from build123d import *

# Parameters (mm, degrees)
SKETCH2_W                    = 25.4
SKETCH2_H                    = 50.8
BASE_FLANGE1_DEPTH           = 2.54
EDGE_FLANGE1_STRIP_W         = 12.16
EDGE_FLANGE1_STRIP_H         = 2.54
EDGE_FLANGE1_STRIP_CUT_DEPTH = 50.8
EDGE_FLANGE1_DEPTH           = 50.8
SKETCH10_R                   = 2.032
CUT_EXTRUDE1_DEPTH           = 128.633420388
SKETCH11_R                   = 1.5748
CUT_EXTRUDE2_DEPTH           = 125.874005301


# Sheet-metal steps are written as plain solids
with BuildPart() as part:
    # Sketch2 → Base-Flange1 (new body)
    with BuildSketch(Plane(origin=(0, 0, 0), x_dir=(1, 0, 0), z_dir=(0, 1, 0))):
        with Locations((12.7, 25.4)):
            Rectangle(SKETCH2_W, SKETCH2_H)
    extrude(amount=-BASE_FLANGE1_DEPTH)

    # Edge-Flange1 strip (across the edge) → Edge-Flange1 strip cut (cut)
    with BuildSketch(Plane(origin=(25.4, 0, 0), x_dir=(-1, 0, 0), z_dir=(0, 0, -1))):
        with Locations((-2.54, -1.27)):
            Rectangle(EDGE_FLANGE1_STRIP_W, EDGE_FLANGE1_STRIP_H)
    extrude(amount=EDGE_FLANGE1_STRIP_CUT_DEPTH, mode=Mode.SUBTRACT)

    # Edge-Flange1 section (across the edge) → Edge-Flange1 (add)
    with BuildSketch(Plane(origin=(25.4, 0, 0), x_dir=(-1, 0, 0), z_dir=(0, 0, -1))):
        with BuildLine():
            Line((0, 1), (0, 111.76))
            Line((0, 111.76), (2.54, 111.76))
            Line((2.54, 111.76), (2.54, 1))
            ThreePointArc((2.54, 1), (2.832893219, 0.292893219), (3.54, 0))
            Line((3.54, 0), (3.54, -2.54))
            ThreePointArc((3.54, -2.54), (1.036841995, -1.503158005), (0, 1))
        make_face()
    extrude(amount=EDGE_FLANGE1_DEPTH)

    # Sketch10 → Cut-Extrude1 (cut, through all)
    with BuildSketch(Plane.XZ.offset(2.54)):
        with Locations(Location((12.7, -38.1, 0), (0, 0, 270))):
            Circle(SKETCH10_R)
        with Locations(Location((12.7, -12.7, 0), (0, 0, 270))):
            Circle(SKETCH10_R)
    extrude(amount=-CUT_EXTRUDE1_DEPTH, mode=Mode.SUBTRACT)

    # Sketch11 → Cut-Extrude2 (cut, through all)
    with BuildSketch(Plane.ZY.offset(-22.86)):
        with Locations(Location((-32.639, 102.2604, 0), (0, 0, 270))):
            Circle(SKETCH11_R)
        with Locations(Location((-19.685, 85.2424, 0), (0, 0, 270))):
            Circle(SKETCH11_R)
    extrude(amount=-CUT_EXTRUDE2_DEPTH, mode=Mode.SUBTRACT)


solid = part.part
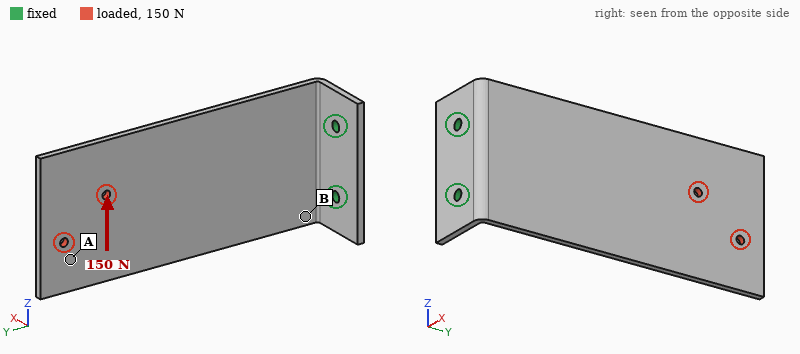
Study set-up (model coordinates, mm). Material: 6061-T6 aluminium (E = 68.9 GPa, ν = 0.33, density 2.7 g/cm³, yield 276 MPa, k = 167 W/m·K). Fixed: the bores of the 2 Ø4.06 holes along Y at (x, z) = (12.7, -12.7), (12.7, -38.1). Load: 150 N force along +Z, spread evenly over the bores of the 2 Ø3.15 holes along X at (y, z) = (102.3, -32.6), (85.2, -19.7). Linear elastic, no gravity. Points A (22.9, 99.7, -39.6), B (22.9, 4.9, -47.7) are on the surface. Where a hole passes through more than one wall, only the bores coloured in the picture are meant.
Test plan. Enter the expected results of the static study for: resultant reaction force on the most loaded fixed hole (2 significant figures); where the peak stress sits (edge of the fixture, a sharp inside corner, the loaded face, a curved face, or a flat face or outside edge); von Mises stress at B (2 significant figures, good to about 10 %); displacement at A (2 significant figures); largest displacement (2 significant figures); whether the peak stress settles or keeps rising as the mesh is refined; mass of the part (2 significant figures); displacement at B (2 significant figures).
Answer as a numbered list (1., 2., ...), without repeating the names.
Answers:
1. 490 N
2. edge of the fixture
3. 52 MPa
4. 0.52 mm
5. 0.59 mm
6. keeps rising
7. 47 g
8. 0.11 mm
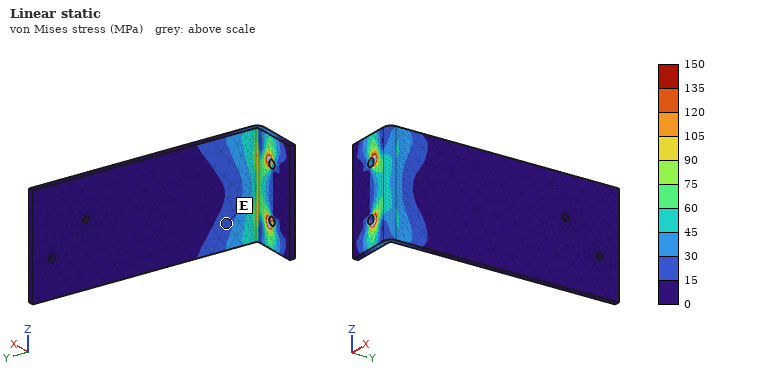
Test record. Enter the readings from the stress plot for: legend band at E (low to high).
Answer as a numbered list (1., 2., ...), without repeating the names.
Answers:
1. 15 to 30 MPa
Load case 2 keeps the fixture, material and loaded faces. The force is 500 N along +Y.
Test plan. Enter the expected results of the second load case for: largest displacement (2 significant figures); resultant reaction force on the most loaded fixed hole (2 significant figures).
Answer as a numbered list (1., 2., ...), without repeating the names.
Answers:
1. 0.78 mm
2. 260 N
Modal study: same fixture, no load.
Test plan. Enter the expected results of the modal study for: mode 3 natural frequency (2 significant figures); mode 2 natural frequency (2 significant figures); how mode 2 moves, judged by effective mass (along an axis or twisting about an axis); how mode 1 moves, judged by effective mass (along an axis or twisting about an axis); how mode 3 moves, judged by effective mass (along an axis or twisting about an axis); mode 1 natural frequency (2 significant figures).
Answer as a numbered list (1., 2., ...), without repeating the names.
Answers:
1. 790 Hz
2. 610 Hz
3. along Z
4. along X
5. along Z
6. 140 Hz
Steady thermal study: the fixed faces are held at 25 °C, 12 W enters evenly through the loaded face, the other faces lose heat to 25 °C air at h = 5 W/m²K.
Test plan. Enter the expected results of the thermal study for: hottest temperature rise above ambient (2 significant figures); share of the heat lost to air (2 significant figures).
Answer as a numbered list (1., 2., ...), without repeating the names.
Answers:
1. 57 K
2. 17 %
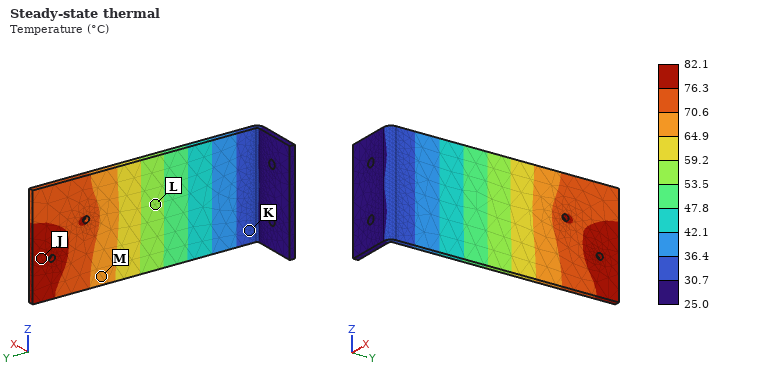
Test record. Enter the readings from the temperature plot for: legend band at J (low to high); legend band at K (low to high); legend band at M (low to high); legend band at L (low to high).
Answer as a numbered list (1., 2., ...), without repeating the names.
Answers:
1. 76.3 to 82.1 °C
2. 30.7 to 36.4 °C
3. 64.9 to 70.6 °C
4. 53.5 to 59.2 °C
